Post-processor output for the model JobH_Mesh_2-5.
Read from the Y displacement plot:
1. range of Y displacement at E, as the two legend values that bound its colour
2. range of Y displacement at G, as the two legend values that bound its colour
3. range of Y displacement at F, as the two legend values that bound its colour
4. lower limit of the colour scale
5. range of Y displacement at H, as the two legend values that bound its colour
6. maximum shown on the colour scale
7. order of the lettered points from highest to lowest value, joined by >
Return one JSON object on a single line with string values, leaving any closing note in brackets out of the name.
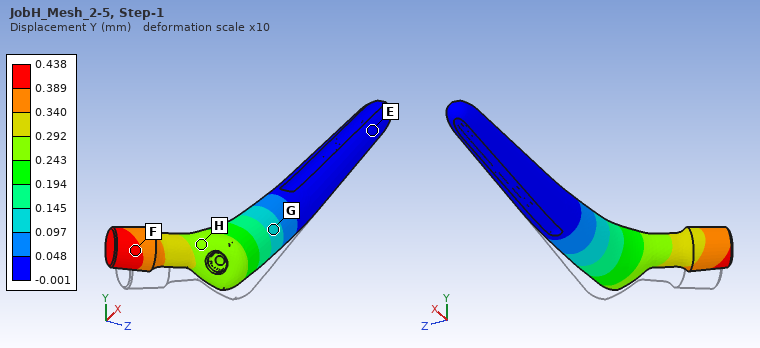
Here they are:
{"range of Y displacement at E, as the two legend values that bound its colour": "-0.001 to 0.048 mm", "range of Y displacement at G, as the two legend values that bound its colour": "0.097 to 0.145 mm", "range of Y displacement at F, as the two legend values that bound its colour": "0.389 to 0.438 mm", "lower limit of the colour scale": "-0.001 mm", "range of Y displacement at H, as the two legend values that bound its colour": "0.243 to 0.292 mm", "maximum shown on the colour scale": "0.438 mm", "order of the lettered points from highest to lowest value, joined by >": "F > H > G > E"}
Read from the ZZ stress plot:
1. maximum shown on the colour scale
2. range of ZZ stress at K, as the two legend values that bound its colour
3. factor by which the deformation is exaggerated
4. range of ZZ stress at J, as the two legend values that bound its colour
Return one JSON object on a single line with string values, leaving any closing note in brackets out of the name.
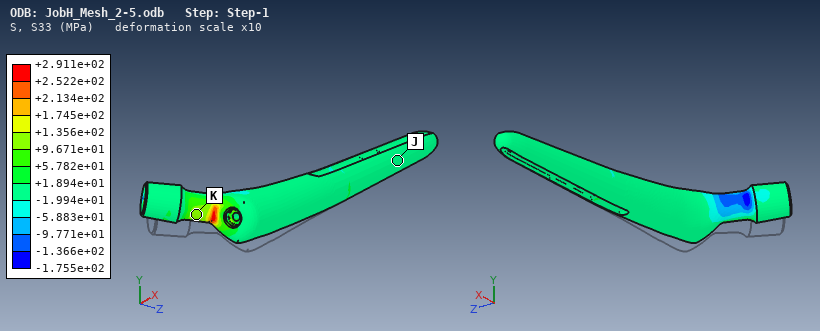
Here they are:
{"maximum shown on the colour scale": "+2.911e+02 MPa", "range of ZZ stress at K, as the two legend values that bound its colour": "+9.671e+01 to +1.356e+02 MPa", "factor by which the deformation is exaggerated": "10", "range of ZZ stress at J, as the two legend values that bound its colour": "-1.994e+01 to +1.894e+01 MPa"}
